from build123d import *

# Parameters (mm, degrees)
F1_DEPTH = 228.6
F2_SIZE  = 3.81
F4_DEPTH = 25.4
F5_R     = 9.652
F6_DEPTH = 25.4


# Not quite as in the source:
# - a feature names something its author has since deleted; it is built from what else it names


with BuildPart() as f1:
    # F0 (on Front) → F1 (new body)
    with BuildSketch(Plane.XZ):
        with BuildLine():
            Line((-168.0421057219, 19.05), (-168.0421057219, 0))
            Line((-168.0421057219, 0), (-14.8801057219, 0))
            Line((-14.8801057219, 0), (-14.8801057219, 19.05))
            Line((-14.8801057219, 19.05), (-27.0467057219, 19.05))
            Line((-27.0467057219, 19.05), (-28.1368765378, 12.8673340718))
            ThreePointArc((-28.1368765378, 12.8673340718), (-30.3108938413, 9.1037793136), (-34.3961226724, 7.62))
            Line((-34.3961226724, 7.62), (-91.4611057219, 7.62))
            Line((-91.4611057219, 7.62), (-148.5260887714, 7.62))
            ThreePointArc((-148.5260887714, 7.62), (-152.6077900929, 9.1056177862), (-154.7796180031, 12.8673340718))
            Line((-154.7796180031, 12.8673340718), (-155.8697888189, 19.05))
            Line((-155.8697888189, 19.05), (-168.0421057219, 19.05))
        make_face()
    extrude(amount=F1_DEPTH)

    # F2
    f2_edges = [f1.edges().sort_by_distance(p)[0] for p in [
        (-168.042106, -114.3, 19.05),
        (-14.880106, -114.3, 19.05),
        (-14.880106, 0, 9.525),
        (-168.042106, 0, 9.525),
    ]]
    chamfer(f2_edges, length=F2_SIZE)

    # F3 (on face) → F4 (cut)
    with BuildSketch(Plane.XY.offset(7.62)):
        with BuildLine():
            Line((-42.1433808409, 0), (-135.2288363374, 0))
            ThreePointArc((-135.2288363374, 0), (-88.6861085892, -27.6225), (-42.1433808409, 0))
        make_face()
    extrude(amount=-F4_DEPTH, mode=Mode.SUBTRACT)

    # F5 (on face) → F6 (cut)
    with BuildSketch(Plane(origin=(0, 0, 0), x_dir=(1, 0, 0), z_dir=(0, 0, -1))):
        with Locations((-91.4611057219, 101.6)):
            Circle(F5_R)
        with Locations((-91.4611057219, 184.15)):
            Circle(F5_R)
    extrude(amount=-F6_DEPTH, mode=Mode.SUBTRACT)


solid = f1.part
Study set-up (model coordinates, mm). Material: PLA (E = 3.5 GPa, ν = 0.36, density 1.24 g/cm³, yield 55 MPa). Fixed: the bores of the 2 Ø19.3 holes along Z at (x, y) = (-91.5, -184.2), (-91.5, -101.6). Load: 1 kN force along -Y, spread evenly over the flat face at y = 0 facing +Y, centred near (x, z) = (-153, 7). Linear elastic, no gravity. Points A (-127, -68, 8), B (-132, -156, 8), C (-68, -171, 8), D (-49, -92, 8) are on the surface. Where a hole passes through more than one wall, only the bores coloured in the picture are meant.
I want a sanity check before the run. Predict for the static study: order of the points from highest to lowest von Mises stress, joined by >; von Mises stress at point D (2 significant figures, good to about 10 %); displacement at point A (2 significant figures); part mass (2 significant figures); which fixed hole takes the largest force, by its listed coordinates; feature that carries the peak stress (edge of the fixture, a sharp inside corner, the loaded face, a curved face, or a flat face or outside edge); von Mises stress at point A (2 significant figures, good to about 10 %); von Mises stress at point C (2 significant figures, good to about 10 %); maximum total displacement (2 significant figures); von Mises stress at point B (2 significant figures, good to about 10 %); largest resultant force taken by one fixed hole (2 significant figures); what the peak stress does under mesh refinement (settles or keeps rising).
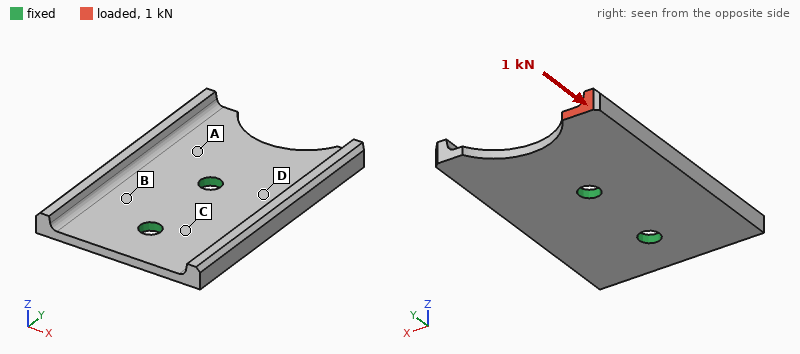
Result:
B > A > C > D
0.48 MPa
0.087 mm
390 g
(-91.5, -101.6)
edge of the fixture
1.5 MPa
0.90 MPa
0.31 mm
2.2 MPa
880 N
keeps rising
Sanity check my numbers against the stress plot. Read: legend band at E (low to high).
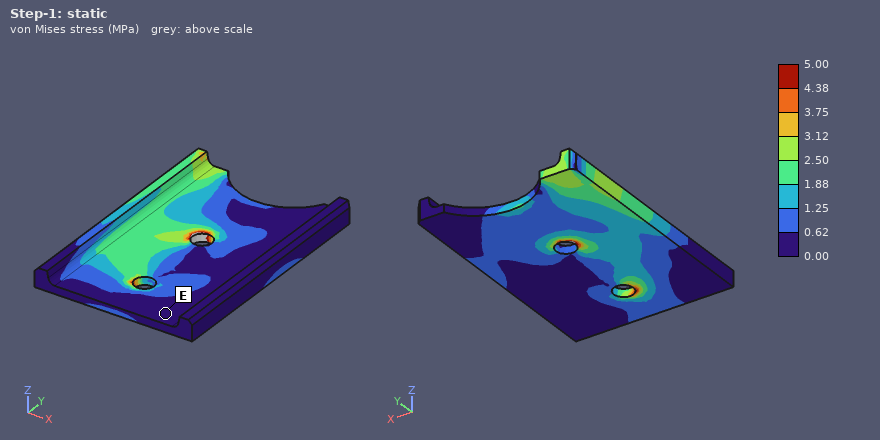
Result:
0.00 to 0.62 MPa
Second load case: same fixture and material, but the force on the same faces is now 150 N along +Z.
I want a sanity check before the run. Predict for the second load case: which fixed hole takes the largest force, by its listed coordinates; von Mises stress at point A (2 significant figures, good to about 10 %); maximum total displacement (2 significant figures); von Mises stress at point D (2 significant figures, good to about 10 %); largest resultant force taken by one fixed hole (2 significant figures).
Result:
(-91.5, -101.6)
3.3 MPa
3.2 mm
1.0 MPa
250 N
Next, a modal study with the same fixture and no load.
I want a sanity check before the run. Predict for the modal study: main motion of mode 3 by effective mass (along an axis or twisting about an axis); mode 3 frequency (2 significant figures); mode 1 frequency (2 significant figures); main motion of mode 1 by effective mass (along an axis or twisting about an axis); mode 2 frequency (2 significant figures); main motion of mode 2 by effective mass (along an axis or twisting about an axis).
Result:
along Z
330 Hz
210 Hz
twisting about Y
230 Hz
along Z
